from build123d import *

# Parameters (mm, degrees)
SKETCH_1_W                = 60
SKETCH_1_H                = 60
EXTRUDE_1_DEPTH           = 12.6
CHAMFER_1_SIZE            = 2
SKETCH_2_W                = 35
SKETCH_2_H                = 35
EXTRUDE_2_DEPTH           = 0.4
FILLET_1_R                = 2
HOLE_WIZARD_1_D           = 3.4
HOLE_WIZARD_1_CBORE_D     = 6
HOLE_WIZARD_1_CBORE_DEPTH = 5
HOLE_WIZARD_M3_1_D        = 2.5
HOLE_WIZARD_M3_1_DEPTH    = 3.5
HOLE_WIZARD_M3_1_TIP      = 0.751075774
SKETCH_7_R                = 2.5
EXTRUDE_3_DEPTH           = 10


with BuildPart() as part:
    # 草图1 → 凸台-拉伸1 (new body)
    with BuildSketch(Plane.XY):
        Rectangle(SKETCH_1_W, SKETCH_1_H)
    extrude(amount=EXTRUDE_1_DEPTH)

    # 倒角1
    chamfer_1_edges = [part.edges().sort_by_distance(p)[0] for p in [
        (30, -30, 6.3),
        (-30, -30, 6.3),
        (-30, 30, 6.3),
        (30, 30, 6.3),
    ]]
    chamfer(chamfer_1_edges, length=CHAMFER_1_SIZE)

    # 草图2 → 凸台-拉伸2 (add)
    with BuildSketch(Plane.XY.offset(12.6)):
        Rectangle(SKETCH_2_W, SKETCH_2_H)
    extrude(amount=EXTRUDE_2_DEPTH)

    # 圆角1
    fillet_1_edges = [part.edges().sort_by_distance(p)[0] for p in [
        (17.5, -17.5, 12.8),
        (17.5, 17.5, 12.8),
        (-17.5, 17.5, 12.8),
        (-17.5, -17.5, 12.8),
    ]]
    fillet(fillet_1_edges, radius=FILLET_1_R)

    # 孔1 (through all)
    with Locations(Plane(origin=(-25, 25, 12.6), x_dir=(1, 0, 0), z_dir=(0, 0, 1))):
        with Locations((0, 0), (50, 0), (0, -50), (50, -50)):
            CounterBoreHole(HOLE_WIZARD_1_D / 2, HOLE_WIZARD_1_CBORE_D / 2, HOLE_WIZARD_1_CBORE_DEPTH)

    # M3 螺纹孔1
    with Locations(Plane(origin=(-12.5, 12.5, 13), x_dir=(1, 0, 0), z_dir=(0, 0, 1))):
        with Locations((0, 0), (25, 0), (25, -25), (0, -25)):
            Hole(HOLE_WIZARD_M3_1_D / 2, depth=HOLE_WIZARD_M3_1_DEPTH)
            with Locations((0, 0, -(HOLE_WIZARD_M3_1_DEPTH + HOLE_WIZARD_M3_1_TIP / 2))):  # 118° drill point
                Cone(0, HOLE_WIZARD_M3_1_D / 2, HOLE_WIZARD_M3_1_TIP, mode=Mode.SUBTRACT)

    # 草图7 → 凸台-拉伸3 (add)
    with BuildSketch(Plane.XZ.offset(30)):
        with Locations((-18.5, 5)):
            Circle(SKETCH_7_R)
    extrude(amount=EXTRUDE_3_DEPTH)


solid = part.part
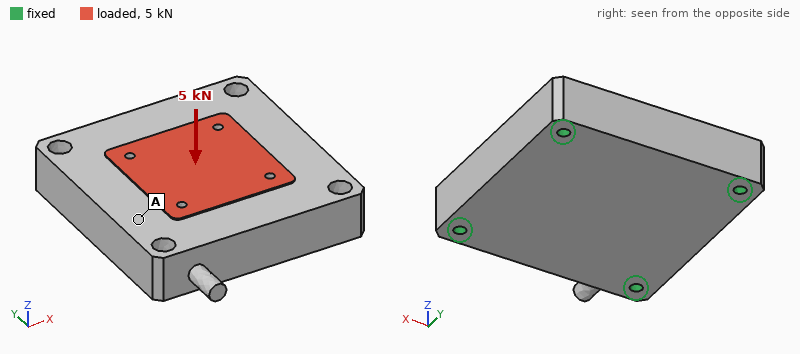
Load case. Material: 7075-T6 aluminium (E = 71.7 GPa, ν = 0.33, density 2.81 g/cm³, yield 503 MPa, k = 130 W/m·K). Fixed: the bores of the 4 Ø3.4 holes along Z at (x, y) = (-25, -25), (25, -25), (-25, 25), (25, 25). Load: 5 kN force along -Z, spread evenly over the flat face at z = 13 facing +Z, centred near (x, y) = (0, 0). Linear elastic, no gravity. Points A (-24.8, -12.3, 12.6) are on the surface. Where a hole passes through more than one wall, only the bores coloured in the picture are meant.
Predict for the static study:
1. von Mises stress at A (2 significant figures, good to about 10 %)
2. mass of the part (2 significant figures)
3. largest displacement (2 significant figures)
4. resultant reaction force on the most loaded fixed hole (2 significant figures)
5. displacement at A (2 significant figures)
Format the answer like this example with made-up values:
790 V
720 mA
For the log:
9.7 MPa
130 g
18 µm
1.5 kN
7.8 µm
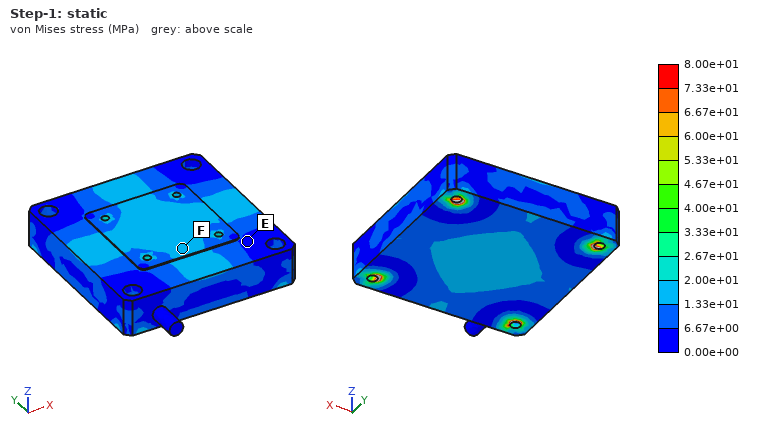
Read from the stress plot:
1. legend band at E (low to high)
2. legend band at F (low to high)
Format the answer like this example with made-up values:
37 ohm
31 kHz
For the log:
0.00e+00 to 6.67e+00 MPa
1.33e+01 to 2.00e+01 MPa
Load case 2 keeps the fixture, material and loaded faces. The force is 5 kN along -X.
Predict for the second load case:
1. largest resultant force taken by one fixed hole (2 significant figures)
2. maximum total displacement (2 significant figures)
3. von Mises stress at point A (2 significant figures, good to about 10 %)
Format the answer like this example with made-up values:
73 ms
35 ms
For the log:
1.5 kN
5.4 µm
4.6 MPa
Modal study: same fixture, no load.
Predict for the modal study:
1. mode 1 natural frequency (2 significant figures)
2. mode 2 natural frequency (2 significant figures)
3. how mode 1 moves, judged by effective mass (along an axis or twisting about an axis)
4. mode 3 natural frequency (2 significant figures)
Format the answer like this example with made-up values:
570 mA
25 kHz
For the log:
11 kHz
17 kHz
along Z
17 kHz
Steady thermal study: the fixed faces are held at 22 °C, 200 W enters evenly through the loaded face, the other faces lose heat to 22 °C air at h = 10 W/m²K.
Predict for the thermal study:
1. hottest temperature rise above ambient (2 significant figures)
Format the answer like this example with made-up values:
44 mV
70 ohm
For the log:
45 K
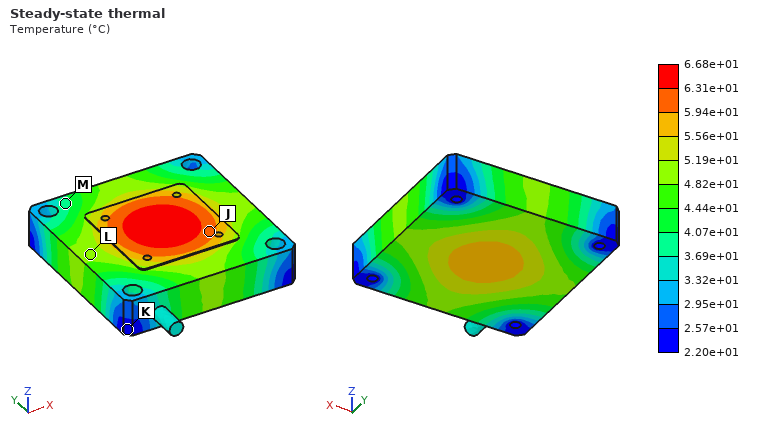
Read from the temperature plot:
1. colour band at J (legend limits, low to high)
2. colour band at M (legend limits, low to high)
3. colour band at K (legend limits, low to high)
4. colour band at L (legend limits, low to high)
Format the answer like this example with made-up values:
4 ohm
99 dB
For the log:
5.94e+01 to 6.31e+01 °C
3.69e+01 to 4.07e+01 °C
2.20e+01 to 2.57e+01 °C
4.82e+01 to 5.19e+01 °C
